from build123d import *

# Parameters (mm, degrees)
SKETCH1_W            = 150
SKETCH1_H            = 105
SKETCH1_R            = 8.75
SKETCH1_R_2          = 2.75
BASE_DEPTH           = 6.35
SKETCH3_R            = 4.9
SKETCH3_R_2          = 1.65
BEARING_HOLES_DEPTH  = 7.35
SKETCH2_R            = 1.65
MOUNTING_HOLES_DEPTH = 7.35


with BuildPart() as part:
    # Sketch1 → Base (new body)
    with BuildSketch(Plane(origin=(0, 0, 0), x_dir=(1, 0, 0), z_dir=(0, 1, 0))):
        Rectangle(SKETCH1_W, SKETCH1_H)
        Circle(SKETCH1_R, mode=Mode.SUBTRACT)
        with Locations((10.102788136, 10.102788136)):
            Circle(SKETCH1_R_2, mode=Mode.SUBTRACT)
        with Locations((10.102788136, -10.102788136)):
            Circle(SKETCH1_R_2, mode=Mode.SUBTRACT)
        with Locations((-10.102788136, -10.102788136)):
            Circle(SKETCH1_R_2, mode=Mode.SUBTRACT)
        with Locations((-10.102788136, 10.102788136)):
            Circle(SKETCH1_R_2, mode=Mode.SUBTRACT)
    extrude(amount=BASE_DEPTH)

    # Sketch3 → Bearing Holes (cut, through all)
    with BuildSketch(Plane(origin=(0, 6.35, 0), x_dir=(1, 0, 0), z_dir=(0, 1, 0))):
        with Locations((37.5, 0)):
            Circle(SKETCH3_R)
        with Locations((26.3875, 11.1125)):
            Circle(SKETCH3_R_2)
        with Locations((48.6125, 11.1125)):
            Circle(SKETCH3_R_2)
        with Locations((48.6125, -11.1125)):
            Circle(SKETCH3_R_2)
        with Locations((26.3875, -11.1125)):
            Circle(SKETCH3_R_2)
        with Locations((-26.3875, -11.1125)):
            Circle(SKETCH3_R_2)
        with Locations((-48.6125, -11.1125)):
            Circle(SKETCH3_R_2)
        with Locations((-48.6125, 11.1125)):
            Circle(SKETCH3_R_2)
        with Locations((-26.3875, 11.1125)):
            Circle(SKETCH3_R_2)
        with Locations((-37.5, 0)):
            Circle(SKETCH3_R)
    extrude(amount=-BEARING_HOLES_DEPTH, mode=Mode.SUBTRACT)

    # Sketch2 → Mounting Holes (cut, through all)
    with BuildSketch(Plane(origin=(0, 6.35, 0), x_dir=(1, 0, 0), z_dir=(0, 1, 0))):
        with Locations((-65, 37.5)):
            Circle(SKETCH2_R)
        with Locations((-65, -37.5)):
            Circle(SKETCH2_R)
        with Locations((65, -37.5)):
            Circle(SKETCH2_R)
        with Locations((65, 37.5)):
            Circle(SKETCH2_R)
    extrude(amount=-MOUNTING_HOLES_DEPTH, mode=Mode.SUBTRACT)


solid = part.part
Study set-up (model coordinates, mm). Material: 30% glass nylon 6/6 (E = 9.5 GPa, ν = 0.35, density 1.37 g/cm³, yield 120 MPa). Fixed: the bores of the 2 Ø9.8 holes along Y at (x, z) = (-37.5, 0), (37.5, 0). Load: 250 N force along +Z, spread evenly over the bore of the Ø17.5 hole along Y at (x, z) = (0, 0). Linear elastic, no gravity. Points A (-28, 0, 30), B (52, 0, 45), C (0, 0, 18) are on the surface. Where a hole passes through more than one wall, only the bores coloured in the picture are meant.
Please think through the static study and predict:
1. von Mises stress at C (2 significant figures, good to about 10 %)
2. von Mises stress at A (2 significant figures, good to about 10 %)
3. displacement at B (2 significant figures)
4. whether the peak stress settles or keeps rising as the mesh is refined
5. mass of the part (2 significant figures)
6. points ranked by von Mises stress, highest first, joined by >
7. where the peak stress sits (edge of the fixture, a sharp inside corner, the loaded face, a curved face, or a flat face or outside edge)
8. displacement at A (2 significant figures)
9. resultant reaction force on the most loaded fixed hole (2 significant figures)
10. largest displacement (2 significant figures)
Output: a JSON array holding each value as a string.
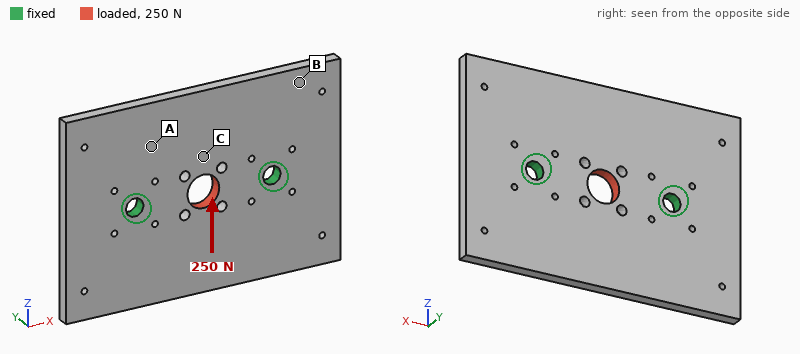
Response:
["0.54 MPa", "0.31 MPa", "0.82 µm", "keeps rising", "130 g", "C > A > B", "edge of the fixture", "1.4 µm", "130 N", "3.9 µm"]
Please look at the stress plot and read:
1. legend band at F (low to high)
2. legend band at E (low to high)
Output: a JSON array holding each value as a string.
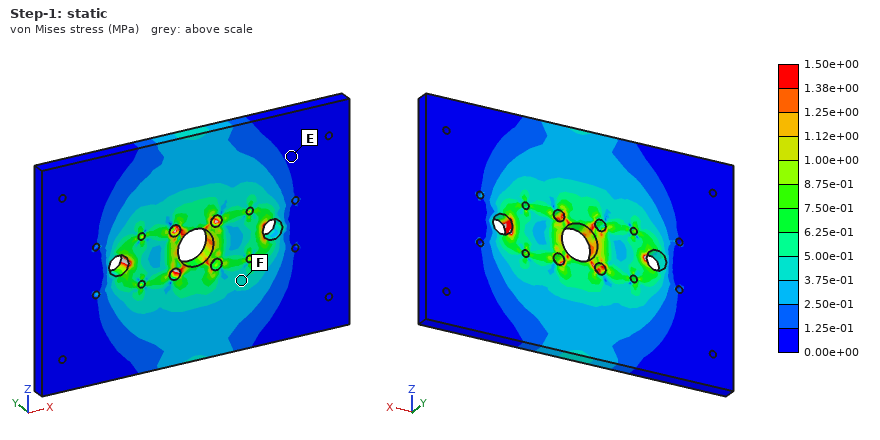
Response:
["3.75e-01 to 5.00e-01 MPa", "0.00e+00 to 1.25e-01 MPa"]
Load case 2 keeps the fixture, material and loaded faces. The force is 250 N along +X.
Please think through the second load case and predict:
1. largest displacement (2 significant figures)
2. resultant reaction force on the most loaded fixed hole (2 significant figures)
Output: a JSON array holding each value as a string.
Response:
["2.8 µm", "130 N"]
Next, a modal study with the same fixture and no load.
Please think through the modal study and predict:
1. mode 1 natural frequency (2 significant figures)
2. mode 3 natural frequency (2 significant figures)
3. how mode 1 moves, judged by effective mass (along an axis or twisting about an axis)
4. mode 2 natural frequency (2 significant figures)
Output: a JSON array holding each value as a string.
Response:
["800 Hz", "1000 Hz", "twisting about X", "990 Hz"]
